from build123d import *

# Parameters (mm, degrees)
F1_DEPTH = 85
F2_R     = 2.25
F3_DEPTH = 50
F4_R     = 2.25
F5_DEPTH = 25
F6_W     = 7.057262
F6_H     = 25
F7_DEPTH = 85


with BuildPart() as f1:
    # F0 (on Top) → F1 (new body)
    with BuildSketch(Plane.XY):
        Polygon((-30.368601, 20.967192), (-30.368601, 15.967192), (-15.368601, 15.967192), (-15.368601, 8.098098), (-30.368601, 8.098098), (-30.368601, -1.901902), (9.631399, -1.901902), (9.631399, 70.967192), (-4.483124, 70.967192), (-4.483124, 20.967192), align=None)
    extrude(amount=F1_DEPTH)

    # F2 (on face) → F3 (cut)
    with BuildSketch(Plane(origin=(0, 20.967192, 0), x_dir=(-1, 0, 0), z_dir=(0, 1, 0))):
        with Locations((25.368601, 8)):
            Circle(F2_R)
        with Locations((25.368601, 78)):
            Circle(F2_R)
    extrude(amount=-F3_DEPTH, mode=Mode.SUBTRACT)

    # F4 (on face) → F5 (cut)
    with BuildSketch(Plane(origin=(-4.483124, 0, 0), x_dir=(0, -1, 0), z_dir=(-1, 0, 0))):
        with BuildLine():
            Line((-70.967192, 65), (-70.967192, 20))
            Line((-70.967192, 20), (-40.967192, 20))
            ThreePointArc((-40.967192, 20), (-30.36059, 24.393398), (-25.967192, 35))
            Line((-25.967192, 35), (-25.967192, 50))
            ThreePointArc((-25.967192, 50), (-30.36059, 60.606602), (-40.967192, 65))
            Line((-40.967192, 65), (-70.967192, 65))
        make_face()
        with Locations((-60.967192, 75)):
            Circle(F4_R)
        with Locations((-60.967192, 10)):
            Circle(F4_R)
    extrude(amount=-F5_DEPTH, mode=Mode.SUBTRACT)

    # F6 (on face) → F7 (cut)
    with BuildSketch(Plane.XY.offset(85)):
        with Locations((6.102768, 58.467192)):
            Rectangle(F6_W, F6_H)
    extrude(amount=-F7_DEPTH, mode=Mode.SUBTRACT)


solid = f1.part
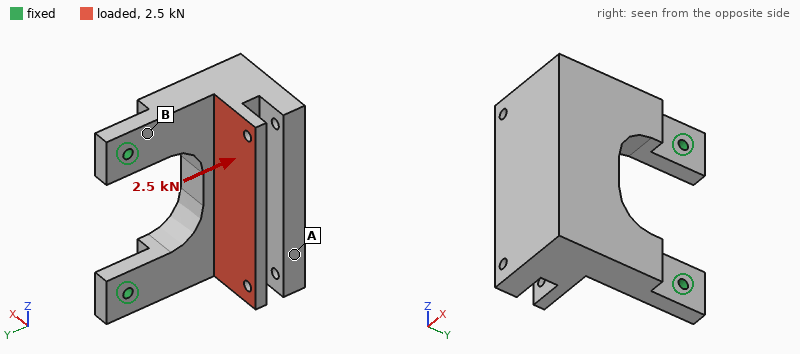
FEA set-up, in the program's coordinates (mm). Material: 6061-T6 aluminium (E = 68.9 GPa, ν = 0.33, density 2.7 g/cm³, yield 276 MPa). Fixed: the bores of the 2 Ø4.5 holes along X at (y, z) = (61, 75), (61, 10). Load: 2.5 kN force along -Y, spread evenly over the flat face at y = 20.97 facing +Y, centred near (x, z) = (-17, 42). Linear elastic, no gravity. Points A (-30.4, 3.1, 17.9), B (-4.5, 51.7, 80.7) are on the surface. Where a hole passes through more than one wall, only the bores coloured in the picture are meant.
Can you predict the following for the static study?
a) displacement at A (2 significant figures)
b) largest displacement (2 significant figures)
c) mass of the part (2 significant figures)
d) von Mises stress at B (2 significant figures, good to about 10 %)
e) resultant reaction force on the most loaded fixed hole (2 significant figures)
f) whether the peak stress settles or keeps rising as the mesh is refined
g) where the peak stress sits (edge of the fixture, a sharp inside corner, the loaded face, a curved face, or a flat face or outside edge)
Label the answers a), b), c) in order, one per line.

a) 0.60 mm
b) 0.64 mm
c) 250 g
d) 120 MPa
e) 1.3 kN
f) keeps rising
g) edge of the fixture
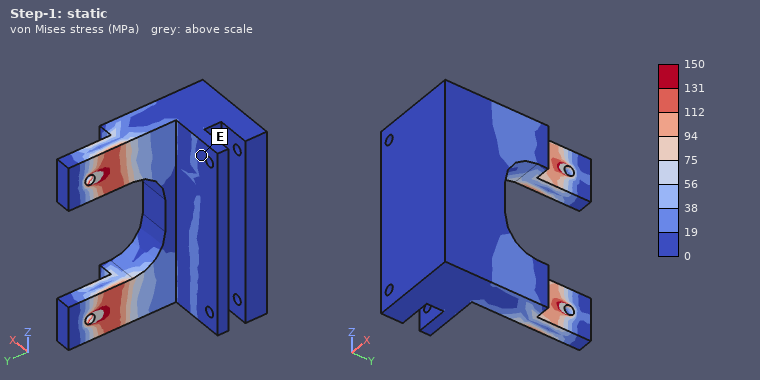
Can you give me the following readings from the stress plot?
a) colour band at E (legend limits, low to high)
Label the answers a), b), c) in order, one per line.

a) 0 to 19 MPa
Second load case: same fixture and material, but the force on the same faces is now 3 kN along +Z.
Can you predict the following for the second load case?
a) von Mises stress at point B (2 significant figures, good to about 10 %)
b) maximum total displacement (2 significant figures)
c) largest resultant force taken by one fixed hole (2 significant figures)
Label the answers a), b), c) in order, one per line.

a) 32 MPa
b) 0.13 mm
c) 2.2 kN
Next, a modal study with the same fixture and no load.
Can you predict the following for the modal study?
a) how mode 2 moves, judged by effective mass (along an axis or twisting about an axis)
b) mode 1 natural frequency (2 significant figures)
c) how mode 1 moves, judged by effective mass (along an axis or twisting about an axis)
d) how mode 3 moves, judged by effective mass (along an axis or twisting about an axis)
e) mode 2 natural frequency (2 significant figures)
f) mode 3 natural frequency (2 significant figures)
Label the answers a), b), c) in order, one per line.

a) along Z
b) 510 Hz
c) along X
d) along Z
e) 2000 Hz
f) 3000 Hz
